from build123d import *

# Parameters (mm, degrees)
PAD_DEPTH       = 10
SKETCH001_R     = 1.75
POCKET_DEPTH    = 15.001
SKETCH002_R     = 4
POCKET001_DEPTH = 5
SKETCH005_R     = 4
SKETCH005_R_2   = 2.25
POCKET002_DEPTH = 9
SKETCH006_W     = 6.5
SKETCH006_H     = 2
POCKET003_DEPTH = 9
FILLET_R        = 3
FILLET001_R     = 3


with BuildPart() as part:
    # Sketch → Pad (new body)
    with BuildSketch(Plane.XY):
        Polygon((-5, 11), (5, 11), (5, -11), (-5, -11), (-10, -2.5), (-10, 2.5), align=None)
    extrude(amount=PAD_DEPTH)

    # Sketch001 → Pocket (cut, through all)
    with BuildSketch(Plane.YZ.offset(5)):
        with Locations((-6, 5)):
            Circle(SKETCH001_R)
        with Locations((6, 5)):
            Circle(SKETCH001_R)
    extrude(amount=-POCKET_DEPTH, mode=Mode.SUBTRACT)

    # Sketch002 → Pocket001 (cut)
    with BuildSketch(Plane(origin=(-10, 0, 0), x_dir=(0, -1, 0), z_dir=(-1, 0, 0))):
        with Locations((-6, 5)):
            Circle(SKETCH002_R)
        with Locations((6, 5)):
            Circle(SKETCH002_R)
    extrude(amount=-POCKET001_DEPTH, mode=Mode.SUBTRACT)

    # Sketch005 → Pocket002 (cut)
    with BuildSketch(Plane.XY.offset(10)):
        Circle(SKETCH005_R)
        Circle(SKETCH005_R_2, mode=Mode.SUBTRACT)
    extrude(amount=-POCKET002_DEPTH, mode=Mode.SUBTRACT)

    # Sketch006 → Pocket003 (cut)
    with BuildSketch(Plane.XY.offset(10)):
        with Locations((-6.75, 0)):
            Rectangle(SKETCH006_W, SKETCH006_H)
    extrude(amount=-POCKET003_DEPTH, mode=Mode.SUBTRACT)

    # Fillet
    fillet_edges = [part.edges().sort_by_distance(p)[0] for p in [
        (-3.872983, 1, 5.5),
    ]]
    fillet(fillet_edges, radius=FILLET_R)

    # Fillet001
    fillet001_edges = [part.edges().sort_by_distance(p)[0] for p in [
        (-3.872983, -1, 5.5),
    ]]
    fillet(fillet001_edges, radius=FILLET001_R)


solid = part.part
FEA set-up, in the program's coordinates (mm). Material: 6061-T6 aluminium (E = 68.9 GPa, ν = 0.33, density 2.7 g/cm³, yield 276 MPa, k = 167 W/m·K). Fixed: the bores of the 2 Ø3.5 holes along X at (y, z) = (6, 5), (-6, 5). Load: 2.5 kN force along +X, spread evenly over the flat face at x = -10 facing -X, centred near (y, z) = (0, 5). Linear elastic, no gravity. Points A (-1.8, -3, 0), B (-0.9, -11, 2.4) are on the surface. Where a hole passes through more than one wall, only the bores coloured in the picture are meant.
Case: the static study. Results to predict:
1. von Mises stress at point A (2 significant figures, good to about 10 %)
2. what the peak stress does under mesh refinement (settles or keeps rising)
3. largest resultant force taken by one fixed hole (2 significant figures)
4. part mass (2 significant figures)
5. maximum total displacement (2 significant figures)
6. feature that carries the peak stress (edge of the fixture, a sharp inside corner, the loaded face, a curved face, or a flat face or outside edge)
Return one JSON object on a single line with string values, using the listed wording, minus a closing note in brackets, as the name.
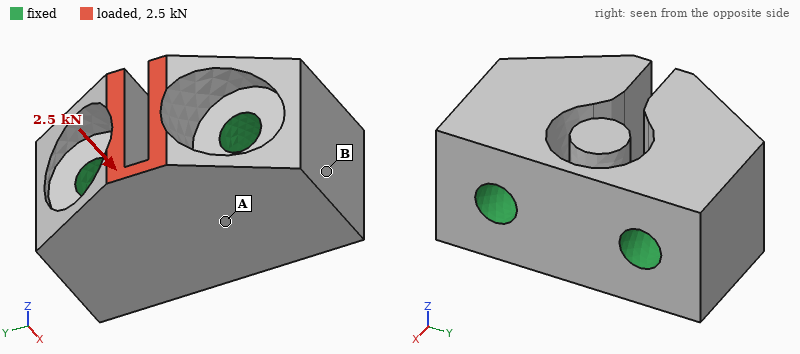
{"von Mises stress at point A": "50 MPa", "what the peak stress does under mesh refinement": "keeps rising", "largest resultant force taken by one fixed hole": "1.3 kN", "part mass": "5.3 g", "maximum total displacement": "28 µm", "feature that carries the peak stress": "edge of the fixture"}
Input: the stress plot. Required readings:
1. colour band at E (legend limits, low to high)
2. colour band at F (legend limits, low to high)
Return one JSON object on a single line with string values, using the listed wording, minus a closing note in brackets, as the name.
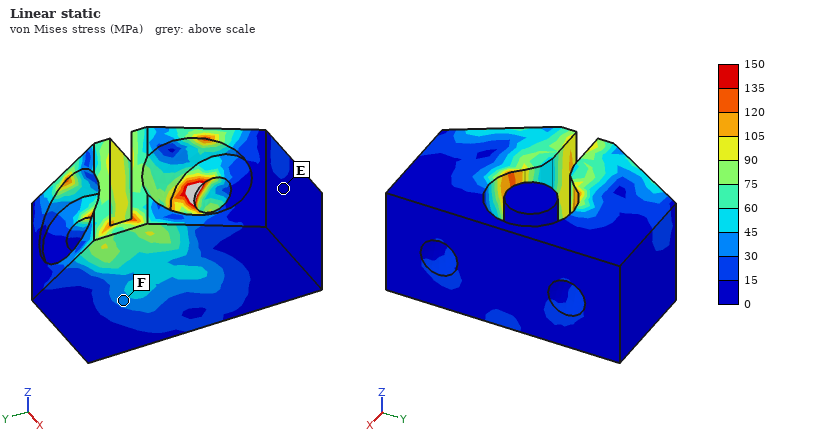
{"colour band at E": "0 to 15 MPa", "colour band at F": "30 to 45 MPa"}
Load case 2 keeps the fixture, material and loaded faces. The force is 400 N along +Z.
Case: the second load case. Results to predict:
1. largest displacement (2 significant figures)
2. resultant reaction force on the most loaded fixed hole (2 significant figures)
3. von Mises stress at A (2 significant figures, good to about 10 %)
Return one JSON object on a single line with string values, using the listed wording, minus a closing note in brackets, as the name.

{"largest displacement": "12 µm", "resultant reaction force on the most loaded fixed hole": "200 N", "von Mises stress at A": "22 MPa"}
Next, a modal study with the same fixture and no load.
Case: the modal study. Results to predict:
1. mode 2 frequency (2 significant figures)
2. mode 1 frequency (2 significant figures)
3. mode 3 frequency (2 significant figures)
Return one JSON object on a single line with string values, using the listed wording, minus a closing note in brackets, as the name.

{"mode 2 frequency": "20 kHz", "mode 1 frequency": "20 kHz", "mode 3 frequency": "50 kHz"}
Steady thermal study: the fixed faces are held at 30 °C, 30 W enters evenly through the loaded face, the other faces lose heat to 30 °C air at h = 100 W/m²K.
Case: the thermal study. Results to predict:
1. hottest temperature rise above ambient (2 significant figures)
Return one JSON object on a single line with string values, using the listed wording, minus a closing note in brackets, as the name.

{"hottest temperature rise above ambient": "32 K"}
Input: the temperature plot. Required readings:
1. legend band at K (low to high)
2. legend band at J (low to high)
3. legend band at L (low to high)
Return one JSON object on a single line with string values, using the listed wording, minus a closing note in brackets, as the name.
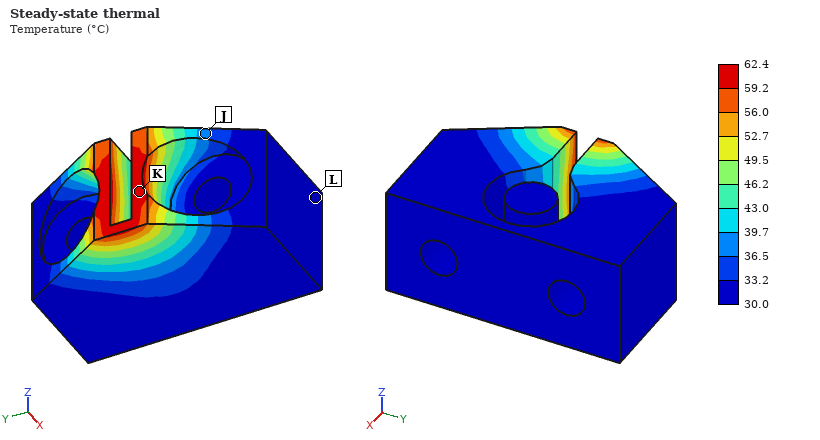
{"legend band at K": "59.2 to 62.4 °C", "legend band at J": "36.5 to 39.7 °C", "legend band at L": "30.0 to 33.2 °C"}
